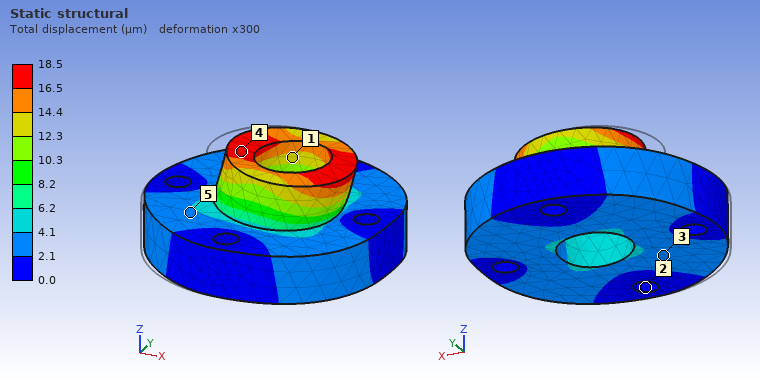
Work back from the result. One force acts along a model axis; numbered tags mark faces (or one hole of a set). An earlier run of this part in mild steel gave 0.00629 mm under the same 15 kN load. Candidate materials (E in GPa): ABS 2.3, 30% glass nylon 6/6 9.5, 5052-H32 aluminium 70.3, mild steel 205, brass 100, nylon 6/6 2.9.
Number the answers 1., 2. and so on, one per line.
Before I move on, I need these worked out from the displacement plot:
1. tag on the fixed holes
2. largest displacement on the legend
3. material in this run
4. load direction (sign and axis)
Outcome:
1. 2
2. 18.5 µm
3. 5052-H32 aluminium
4. +X
